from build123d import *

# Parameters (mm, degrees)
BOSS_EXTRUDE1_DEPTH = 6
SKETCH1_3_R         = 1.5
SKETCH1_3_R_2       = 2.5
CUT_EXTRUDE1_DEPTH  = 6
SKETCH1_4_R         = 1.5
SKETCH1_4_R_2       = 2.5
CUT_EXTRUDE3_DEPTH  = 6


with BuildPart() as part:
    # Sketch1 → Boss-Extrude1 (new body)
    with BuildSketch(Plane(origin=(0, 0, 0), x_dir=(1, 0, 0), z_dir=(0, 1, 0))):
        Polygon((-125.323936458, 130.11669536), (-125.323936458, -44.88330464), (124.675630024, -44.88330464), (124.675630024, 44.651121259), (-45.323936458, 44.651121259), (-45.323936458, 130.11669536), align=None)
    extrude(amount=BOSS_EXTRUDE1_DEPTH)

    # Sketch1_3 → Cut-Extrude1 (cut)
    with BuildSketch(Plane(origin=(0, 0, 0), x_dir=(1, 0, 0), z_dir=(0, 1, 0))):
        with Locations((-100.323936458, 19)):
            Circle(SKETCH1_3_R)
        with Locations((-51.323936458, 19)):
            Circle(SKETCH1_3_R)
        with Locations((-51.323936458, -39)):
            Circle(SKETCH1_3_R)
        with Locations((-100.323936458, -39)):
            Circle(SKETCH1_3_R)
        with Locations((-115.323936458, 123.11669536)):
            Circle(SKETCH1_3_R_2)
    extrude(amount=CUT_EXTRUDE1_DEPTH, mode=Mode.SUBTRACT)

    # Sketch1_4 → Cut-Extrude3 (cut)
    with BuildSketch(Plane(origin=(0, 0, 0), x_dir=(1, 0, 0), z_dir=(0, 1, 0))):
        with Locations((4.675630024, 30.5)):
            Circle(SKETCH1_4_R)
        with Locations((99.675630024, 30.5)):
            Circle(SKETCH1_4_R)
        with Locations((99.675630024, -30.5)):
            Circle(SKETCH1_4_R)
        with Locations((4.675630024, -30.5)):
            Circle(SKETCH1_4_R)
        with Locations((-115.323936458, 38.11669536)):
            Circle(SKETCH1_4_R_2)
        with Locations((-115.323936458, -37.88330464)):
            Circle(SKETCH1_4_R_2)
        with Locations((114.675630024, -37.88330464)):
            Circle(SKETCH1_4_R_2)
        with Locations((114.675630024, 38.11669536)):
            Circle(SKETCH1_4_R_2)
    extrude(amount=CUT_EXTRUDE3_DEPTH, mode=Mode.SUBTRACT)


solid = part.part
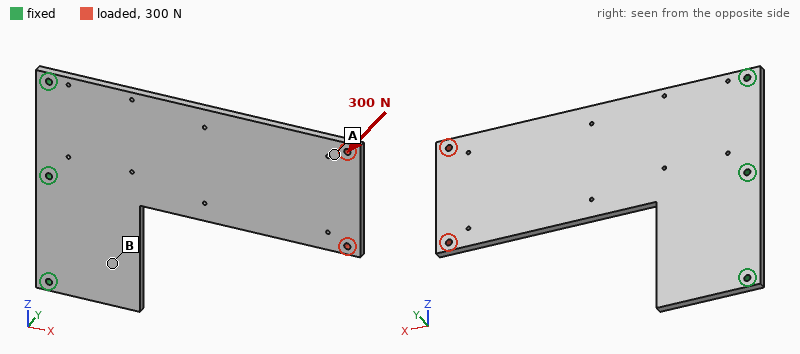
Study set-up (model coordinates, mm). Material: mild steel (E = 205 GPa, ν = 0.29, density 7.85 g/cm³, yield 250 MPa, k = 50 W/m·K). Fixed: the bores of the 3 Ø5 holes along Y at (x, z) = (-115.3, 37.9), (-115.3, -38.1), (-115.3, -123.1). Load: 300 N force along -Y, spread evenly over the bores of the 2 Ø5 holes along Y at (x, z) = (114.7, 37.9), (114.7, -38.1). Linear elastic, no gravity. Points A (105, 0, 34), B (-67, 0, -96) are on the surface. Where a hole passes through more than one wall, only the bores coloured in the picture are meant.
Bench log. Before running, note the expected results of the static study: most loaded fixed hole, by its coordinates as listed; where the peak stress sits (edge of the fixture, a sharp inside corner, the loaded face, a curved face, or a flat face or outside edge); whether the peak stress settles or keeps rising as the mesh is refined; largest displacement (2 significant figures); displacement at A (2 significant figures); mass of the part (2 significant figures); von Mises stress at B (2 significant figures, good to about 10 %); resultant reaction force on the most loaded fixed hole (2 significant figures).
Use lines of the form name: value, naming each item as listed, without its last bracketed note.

most loaded fixed hole, by its coordinates as listed: (-115.3, -38.1)
where the peak stress sits: edge of the fixture
whether the peak stress settles or keeps rising as the mesh is refined: keeps rising
largest displacement: 3.6 mm
displacement at A: 3.1 mm
mass of the part: 1.4 kg
von Mises stress at B: 30 MPa
resultant reaction force on the most loaded fixed hole: 310 N
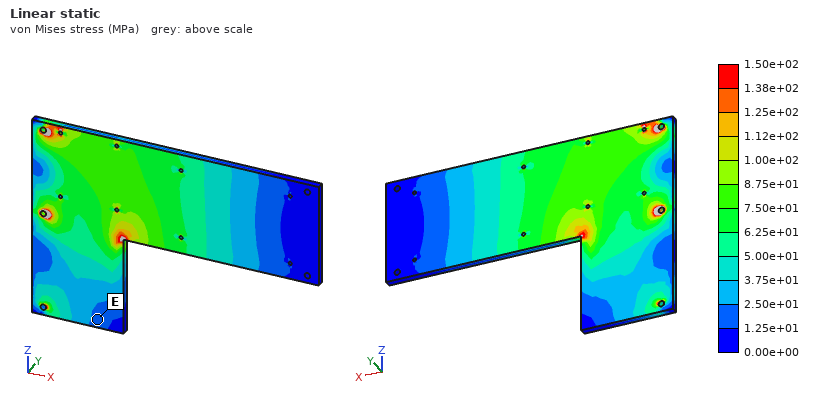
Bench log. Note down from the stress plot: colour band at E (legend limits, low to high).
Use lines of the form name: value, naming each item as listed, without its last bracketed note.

colour band at E: 1.25e+01 to 2.50e+01 MPa
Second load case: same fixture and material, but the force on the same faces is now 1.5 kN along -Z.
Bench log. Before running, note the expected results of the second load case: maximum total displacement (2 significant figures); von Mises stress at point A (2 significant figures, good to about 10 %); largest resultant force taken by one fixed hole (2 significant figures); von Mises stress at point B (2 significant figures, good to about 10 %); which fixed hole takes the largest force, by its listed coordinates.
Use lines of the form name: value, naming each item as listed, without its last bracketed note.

maximum total displacement: 76 µm
von Mises stress at point A: 5.9 MPa
largest resultant force taken by one fixed hole: 3.0 kN
von Mises stress at point B: 5.3 MPa
which fixed hole takes the largest force, by its listed coordinates: (-115.3, 37.9)
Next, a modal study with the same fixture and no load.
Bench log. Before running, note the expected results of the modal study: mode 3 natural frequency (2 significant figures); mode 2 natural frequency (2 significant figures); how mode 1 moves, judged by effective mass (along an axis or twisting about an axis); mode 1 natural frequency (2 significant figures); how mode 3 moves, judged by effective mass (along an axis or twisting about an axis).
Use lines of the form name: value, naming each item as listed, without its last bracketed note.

mode 3 natural frequency: 540 Hz
mode 2 natural frequency: 500 Hz
how mode 1 moves, judged by effective mass: along Y
mode 1 natural frequency: 92 Hz
how mode 3 moves, judged by effective mass: along Y
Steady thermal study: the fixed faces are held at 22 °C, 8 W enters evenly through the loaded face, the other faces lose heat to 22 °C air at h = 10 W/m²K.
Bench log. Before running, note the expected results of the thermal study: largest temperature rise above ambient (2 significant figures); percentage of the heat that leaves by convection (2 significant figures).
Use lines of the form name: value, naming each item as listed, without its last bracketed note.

largest temperature rise above ambient: 37 K
percentage of the heat that leaves by convection: 76 %
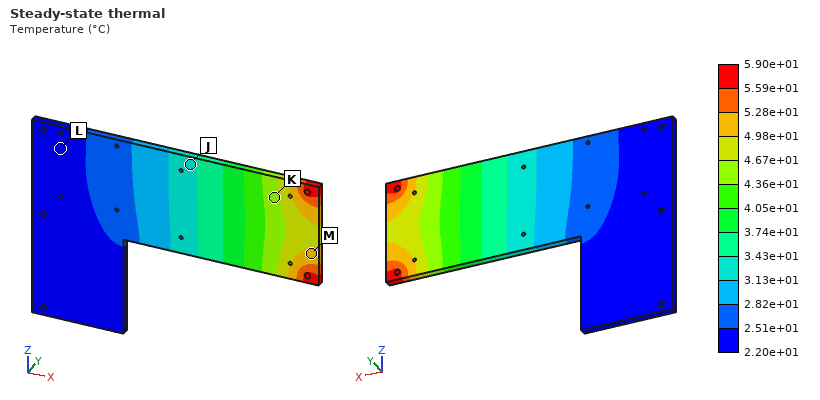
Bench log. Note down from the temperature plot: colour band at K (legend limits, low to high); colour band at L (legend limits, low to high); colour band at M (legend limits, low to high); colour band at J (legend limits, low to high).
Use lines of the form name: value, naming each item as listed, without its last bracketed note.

colour band at K: 4.36e+01 to 4.67e+01 °C
colour band at L: 2.20e+01 to 2.51e+01 °C
colour band at M: 4.98e+01 to 5.28e+01 °C
colour band at J: 3.13e+01 to 3.43e+01 °C
